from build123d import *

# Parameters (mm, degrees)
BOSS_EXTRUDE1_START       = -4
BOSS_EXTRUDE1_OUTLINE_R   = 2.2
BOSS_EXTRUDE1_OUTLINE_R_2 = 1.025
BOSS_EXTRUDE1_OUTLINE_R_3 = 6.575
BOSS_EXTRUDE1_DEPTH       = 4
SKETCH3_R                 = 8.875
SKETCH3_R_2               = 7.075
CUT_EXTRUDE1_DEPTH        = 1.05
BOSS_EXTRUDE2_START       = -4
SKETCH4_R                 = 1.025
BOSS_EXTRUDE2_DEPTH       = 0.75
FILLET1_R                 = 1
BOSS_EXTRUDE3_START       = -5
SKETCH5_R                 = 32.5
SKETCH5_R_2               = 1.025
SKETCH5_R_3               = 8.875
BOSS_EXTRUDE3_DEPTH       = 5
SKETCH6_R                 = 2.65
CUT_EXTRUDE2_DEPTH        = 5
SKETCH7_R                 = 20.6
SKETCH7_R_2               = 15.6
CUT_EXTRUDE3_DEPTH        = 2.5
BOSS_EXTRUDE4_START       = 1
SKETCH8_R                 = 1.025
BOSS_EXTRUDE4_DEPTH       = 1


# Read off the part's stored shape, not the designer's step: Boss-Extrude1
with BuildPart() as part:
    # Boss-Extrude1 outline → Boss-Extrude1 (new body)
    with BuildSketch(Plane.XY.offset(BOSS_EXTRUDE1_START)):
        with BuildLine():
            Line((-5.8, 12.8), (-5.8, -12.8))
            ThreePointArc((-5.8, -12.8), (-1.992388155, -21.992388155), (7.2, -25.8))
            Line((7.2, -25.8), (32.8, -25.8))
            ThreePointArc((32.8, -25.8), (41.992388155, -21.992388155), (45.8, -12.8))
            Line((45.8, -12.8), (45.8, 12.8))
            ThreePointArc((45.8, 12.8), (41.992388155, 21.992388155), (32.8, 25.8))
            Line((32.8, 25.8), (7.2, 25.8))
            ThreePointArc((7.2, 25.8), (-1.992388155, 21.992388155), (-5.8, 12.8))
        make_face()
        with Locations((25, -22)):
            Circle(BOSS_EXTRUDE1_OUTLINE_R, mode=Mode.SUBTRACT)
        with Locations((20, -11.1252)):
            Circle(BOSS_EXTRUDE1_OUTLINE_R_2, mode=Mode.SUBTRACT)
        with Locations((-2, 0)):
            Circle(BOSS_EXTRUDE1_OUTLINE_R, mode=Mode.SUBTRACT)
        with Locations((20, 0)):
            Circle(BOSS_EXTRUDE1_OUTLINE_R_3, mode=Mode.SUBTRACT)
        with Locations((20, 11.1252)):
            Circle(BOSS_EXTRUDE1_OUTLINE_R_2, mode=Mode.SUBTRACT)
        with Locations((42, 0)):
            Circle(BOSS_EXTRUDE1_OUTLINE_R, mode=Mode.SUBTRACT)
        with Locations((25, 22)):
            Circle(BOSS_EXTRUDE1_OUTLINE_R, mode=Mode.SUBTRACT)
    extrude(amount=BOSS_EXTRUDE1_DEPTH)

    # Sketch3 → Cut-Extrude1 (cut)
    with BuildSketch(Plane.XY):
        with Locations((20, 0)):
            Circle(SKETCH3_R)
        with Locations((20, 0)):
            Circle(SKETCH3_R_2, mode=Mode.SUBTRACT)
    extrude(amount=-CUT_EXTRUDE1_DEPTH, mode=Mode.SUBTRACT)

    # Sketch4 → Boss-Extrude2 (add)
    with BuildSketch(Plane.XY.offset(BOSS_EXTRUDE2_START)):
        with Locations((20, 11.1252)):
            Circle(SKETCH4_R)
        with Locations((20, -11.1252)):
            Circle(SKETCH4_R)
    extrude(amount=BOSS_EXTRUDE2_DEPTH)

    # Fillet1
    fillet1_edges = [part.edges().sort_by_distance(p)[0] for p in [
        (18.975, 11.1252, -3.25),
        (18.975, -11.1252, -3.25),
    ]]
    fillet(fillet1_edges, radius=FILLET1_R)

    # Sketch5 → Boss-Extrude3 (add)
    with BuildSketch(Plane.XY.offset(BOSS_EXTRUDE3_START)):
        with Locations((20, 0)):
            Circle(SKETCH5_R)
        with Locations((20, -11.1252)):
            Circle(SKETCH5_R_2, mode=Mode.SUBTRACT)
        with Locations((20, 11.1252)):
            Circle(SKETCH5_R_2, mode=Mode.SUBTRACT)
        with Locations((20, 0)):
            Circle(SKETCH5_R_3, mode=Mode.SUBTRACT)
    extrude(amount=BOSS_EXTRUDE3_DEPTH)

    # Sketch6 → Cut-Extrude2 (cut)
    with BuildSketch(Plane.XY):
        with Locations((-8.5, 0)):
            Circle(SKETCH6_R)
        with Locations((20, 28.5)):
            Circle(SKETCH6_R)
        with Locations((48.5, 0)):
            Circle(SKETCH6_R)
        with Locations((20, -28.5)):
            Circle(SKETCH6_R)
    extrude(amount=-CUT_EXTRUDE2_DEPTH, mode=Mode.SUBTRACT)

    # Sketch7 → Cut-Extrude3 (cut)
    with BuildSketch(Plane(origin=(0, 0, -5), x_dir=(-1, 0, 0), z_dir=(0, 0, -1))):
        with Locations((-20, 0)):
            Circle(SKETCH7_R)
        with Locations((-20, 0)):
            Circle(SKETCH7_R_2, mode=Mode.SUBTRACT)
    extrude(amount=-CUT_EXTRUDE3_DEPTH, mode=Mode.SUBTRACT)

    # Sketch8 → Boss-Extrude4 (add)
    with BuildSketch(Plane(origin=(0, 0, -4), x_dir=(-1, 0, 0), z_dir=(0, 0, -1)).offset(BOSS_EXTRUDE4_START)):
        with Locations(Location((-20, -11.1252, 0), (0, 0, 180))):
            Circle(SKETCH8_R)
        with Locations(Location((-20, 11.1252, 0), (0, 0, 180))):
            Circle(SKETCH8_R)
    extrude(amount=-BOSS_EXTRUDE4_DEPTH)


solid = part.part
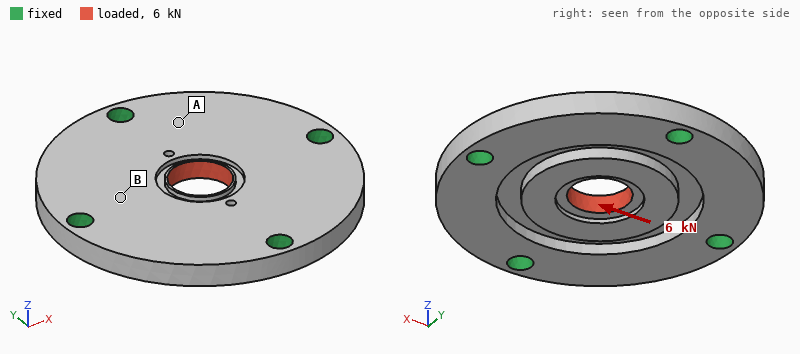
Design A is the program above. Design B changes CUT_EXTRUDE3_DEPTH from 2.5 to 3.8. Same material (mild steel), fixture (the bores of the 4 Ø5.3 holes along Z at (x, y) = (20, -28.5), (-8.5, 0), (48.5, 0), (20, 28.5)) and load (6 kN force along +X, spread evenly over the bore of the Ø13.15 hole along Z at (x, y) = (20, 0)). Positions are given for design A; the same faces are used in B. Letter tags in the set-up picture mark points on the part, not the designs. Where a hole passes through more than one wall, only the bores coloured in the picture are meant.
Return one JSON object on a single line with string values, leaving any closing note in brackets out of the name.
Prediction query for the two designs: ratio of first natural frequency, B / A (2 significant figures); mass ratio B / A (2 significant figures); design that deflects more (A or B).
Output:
{"ratio of first natural frequency, B / A": "0.84", "mass ratio B / A": "0.95", "design that deflects more": "B"}
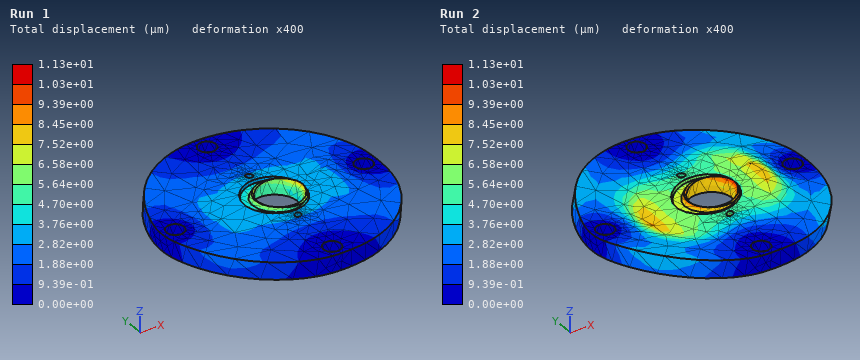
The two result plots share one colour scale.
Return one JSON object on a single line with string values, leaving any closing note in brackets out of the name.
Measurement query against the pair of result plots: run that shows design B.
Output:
{"run that shows design B": "Run 2"}
